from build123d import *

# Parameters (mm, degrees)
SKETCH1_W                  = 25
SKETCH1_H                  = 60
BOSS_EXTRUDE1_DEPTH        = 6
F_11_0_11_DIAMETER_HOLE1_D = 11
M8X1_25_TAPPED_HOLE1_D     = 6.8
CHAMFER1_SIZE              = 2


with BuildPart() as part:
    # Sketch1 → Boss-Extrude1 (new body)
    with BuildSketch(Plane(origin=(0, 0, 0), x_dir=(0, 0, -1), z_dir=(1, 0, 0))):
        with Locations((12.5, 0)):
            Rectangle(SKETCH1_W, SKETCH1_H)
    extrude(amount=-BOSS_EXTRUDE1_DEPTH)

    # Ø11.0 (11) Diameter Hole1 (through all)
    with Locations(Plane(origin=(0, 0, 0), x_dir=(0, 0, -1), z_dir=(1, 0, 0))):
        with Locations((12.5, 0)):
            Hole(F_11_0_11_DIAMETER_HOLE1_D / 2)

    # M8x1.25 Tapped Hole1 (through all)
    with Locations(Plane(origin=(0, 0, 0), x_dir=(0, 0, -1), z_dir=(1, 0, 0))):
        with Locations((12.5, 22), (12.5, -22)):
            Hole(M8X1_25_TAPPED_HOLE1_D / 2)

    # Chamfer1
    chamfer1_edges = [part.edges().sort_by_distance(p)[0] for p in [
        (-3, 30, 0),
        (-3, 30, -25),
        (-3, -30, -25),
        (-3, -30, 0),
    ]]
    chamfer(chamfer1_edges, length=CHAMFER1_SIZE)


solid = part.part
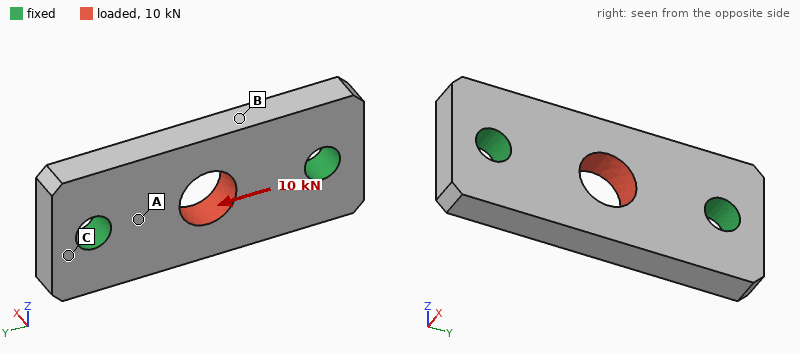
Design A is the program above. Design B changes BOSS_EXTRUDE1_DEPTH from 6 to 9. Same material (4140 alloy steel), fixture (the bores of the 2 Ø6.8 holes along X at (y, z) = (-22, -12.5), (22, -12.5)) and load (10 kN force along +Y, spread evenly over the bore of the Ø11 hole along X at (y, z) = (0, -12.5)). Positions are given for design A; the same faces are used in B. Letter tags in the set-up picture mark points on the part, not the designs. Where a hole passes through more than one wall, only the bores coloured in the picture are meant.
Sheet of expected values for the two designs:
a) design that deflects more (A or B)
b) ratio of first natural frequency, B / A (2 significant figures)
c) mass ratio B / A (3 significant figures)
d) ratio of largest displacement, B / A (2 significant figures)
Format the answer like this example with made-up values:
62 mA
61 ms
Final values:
A
1.3
1.50
0.67
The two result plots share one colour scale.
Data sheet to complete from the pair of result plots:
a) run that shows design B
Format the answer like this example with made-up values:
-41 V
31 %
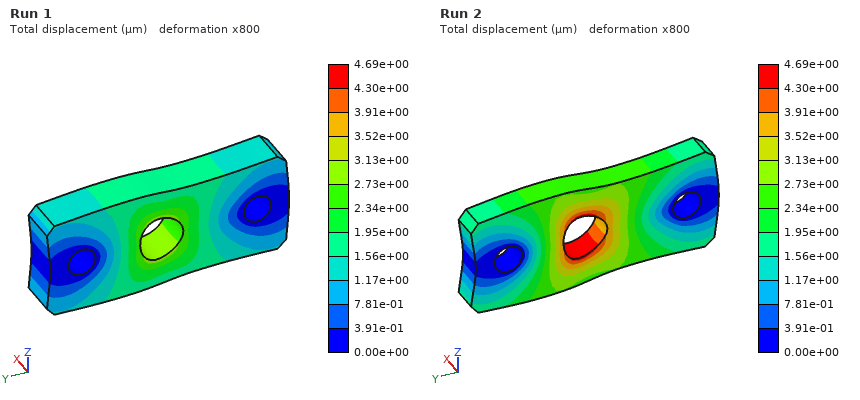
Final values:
Run 1
